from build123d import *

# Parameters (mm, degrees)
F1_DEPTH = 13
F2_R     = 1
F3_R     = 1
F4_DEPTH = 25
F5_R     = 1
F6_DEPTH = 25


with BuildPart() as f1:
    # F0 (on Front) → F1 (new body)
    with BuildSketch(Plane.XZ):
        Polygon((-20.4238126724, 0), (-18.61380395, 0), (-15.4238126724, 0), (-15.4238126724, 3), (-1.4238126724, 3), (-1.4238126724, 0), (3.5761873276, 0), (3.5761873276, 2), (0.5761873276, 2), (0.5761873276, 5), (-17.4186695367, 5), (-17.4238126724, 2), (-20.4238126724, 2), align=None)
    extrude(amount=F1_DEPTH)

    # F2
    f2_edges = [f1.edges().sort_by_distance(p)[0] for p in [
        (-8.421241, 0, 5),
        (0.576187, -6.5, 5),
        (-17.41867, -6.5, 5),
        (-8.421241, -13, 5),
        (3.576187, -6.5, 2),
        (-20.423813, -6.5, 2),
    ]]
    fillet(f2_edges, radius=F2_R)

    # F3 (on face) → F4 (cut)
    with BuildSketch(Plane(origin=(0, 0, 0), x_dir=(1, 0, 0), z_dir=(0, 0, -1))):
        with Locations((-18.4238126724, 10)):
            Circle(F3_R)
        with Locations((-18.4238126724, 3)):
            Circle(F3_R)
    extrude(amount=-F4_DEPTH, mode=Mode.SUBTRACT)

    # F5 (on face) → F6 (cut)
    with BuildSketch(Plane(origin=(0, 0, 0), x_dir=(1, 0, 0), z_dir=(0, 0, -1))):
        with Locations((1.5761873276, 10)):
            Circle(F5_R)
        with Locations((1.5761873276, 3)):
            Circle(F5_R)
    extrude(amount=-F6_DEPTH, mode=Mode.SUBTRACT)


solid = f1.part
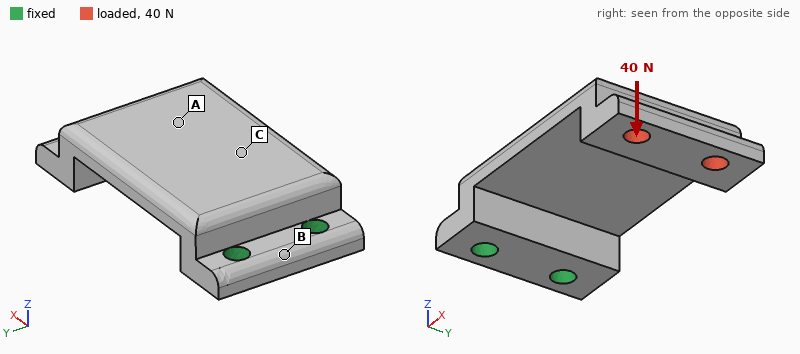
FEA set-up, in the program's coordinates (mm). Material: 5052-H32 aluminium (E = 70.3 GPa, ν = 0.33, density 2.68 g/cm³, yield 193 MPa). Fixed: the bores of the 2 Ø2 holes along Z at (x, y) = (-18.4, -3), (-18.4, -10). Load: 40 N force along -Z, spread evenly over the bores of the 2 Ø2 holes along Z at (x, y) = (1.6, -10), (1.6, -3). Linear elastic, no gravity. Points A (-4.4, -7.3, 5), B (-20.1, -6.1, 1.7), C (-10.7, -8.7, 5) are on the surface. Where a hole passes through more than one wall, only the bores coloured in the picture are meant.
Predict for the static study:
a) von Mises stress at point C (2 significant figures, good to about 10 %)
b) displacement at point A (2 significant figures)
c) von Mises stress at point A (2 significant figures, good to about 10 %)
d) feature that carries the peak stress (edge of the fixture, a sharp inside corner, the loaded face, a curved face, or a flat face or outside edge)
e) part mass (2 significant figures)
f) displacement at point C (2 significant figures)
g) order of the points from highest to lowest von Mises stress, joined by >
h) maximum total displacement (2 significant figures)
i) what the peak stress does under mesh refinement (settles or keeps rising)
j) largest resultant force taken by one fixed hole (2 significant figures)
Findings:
54 MPa
0.12 mm
27 MPa
edge of the fixture
2.0 g
0.046 mm
C > A > B
0.23 mm
keeps rising
24 N
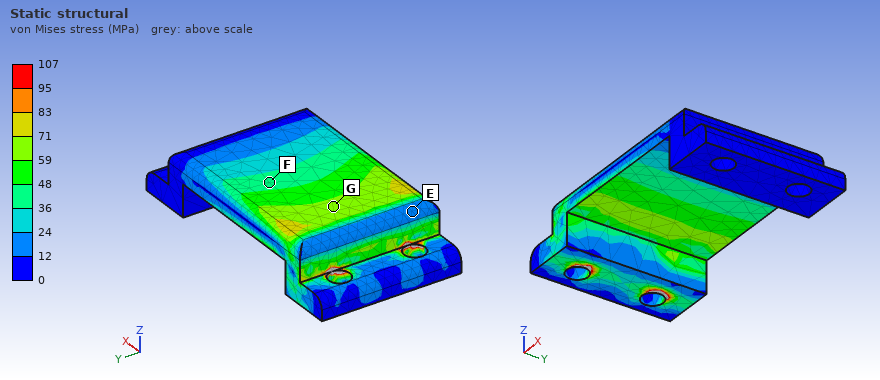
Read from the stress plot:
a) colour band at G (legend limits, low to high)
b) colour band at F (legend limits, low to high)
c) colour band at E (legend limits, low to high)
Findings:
59 to 71 MPa
36 to 48 MPa
12 to 24 MPa
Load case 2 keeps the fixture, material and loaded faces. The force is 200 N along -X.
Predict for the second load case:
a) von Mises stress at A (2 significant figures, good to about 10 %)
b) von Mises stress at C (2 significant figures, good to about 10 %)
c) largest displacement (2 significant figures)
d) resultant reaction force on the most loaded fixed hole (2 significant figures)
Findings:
57 MPa
58 MPa
0.22 mm
100 N
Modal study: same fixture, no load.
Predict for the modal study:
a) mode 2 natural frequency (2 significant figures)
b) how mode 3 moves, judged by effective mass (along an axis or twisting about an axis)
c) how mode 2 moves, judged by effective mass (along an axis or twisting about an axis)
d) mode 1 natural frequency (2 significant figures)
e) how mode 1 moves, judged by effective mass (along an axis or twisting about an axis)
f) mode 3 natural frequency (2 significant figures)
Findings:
7800 Hz
along Y
along Y
2900 Hz
along Z
14 kHz
